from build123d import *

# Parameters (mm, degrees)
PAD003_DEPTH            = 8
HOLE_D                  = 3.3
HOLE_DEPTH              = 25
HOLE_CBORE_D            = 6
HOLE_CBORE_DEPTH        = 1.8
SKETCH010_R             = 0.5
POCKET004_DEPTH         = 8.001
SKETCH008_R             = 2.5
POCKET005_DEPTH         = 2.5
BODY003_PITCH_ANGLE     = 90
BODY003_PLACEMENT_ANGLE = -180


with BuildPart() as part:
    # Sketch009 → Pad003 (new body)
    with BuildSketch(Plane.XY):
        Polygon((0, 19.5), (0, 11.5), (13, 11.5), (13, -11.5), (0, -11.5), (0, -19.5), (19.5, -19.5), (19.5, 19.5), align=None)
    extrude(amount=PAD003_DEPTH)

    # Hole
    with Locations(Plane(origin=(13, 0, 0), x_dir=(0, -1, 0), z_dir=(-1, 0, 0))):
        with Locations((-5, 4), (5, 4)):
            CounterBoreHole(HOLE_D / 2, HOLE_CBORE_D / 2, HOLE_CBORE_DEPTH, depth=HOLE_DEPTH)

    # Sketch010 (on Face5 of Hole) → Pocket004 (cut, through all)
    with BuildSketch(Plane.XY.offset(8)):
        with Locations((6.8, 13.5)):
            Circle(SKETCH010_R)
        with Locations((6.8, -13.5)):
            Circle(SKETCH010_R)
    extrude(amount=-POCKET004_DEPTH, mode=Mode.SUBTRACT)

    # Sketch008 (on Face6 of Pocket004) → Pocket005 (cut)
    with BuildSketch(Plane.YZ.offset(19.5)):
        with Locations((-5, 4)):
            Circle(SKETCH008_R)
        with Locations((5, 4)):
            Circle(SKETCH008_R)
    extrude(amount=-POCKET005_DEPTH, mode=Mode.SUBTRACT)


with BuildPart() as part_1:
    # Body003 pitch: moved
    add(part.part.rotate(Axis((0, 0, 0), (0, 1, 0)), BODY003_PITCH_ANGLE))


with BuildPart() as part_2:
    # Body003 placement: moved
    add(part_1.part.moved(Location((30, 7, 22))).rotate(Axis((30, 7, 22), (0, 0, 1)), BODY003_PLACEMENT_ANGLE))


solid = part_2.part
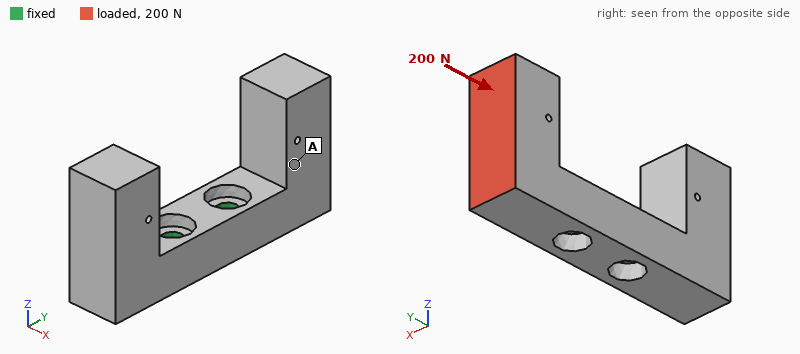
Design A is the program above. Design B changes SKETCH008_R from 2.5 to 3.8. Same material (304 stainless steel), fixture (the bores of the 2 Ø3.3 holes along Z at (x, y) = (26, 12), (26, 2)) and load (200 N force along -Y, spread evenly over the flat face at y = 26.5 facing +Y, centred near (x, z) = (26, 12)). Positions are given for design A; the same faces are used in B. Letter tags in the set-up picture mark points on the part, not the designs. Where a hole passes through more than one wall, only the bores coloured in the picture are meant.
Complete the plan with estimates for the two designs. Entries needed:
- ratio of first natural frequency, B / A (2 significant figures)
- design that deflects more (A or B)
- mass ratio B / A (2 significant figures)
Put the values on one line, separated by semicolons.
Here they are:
0.82; B; 0.96
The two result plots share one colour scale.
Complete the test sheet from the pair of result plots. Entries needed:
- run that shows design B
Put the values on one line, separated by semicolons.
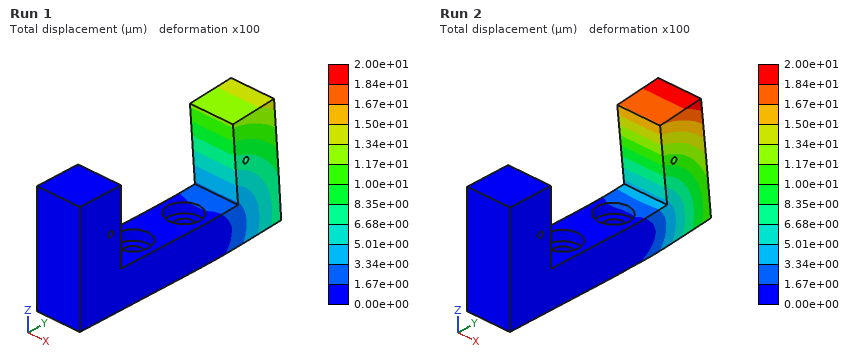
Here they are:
Run 2
